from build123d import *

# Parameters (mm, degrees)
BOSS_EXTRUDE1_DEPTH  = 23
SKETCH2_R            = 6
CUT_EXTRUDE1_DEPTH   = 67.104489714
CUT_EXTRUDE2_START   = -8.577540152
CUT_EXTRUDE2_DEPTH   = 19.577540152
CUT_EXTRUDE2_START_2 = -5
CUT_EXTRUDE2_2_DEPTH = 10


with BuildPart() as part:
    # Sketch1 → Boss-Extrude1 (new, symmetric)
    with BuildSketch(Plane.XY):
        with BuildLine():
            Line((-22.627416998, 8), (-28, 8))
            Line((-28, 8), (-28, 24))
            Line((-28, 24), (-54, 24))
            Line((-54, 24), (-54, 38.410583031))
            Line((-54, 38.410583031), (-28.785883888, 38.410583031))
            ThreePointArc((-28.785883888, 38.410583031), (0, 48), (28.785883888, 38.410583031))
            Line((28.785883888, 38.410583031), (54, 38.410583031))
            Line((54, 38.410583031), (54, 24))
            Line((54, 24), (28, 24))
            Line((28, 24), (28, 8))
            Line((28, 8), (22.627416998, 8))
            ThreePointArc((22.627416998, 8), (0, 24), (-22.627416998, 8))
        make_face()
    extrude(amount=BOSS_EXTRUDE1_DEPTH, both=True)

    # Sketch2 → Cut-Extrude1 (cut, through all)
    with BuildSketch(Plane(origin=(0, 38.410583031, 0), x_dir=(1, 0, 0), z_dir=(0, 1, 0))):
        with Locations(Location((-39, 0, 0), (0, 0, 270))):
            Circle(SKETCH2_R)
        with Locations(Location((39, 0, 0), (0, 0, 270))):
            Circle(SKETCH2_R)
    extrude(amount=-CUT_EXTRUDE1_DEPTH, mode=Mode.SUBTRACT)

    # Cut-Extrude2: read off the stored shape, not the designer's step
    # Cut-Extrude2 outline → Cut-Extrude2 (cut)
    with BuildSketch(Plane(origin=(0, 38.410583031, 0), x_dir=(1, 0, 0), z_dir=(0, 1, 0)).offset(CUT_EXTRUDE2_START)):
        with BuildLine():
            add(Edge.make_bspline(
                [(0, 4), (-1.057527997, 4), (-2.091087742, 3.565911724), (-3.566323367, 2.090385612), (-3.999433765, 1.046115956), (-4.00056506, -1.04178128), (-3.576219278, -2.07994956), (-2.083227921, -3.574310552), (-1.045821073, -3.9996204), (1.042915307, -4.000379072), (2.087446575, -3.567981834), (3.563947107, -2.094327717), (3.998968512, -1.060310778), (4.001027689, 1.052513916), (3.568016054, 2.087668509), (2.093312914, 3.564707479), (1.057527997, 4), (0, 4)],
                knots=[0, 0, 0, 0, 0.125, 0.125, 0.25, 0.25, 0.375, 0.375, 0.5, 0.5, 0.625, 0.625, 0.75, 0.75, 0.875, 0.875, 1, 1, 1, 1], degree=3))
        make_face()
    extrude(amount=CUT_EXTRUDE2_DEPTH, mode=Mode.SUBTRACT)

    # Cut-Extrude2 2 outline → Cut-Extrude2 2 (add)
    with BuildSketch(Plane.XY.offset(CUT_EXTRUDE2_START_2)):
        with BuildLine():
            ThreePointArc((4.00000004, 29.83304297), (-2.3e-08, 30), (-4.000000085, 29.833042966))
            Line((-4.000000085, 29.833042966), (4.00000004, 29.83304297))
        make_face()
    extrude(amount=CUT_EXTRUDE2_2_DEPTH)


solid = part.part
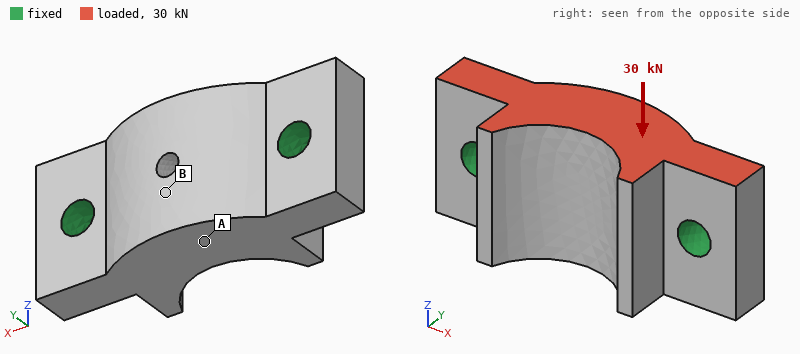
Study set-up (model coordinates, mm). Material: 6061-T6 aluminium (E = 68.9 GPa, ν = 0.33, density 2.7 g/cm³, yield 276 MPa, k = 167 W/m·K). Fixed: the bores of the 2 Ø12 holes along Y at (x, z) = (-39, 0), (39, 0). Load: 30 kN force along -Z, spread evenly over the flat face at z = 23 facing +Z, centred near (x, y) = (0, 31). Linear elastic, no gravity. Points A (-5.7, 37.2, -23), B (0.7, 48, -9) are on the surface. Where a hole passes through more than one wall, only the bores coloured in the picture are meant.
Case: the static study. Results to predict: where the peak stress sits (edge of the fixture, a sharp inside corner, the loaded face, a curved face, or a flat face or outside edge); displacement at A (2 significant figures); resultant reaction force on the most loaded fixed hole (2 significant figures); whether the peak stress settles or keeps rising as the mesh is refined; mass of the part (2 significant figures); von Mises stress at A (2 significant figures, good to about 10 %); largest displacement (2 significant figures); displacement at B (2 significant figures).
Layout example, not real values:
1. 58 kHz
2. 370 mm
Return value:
1. edge of the fixture
2. 17 µm
3. 15 kN
4. keeps rising
5. 270 g
6. 20 MPa
7. 25 µm
8. 19 µm
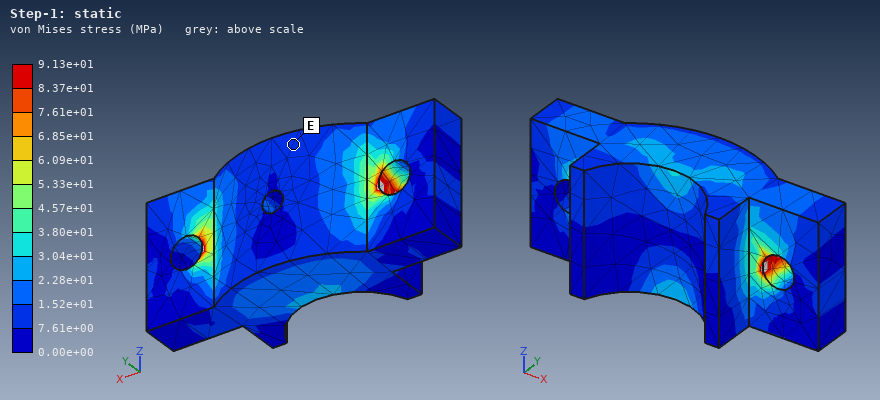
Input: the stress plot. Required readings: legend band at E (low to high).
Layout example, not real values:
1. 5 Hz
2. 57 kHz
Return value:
1. 7.61e+00 to 1.52e+01 MPa
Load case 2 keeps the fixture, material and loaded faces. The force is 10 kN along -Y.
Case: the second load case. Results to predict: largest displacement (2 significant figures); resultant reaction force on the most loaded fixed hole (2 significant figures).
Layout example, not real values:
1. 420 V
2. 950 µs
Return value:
1. 49 µm
2. 5.0 kN
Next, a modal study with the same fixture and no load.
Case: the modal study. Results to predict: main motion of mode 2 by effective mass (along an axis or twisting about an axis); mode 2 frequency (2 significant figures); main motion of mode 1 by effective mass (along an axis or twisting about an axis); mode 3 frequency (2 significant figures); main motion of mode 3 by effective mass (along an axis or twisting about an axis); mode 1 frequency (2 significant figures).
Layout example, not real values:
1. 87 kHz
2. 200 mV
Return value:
1. along Y
2. 10000 Hz
3. twisting about X
4. 12 kHz
5. along Z
6. 8700 Hz
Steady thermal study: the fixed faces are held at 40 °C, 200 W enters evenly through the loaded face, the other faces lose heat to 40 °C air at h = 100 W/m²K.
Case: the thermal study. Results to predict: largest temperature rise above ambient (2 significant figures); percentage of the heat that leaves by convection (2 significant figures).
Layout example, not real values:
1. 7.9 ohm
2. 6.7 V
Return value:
1. 22 K
2. 6.9 %
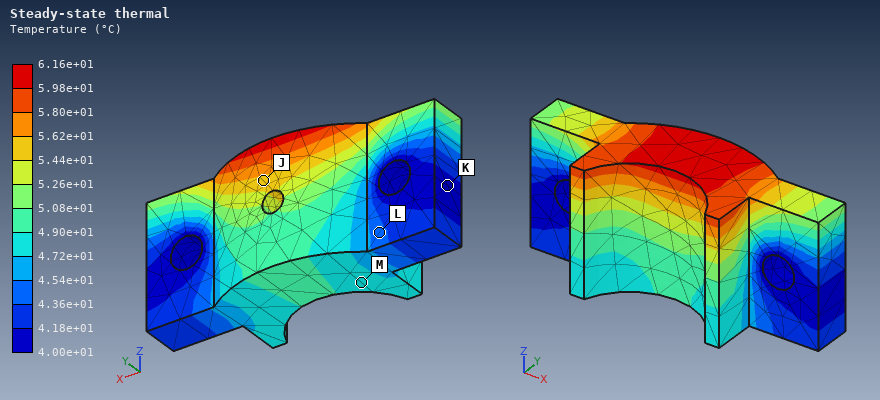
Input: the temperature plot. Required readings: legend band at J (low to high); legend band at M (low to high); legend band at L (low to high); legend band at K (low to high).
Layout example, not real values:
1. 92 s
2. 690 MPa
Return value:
1. 5.44e+01 to 5.62e+01 °C
2. 4.72e+01 to 4.90e+01 °C
3. 4.36e+01 to 4.54e+01 °C
4. 4.00e+01 to 4.18e+01 °C
